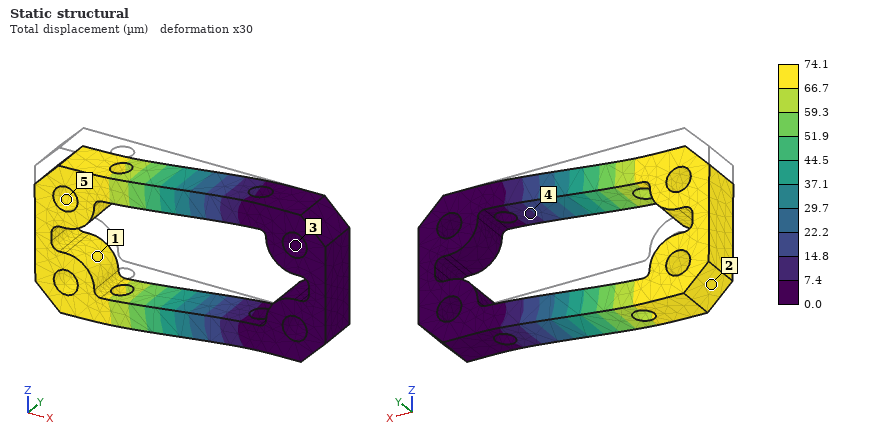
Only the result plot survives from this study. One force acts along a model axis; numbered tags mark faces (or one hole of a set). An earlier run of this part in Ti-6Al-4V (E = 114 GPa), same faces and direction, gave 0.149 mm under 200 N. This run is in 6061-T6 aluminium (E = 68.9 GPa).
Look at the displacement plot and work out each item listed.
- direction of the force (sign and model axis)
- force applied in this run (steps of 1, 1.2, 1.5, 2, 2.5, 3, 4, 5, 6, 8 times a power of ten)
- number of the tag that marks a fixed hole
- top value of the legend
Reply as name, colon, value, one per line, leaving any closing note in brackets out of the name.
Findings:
direction of the force: -Z
force applied in this run: 60 N
number of the tag that marks a fixed hole: 3
top value of the legend: 74.1 µm
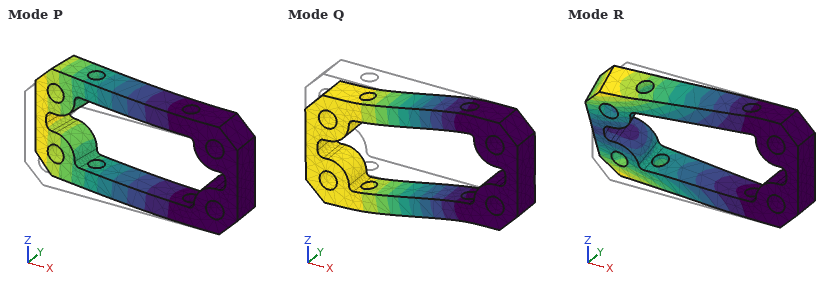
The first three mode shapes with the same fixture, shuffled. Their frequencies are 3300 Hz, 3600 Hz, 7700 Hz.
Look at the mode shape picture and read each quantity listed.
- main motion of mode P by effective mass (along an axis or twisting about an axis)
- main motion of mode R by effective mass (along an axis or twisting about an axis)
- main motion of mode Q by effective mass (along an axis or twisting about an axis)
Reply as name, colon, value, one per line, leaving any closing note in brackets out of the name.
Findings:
main motion of mode P by effective mass: along Y
main motion of mode R by effective mass: twisting about X
main motion of mode Q by effective mass: along Z
